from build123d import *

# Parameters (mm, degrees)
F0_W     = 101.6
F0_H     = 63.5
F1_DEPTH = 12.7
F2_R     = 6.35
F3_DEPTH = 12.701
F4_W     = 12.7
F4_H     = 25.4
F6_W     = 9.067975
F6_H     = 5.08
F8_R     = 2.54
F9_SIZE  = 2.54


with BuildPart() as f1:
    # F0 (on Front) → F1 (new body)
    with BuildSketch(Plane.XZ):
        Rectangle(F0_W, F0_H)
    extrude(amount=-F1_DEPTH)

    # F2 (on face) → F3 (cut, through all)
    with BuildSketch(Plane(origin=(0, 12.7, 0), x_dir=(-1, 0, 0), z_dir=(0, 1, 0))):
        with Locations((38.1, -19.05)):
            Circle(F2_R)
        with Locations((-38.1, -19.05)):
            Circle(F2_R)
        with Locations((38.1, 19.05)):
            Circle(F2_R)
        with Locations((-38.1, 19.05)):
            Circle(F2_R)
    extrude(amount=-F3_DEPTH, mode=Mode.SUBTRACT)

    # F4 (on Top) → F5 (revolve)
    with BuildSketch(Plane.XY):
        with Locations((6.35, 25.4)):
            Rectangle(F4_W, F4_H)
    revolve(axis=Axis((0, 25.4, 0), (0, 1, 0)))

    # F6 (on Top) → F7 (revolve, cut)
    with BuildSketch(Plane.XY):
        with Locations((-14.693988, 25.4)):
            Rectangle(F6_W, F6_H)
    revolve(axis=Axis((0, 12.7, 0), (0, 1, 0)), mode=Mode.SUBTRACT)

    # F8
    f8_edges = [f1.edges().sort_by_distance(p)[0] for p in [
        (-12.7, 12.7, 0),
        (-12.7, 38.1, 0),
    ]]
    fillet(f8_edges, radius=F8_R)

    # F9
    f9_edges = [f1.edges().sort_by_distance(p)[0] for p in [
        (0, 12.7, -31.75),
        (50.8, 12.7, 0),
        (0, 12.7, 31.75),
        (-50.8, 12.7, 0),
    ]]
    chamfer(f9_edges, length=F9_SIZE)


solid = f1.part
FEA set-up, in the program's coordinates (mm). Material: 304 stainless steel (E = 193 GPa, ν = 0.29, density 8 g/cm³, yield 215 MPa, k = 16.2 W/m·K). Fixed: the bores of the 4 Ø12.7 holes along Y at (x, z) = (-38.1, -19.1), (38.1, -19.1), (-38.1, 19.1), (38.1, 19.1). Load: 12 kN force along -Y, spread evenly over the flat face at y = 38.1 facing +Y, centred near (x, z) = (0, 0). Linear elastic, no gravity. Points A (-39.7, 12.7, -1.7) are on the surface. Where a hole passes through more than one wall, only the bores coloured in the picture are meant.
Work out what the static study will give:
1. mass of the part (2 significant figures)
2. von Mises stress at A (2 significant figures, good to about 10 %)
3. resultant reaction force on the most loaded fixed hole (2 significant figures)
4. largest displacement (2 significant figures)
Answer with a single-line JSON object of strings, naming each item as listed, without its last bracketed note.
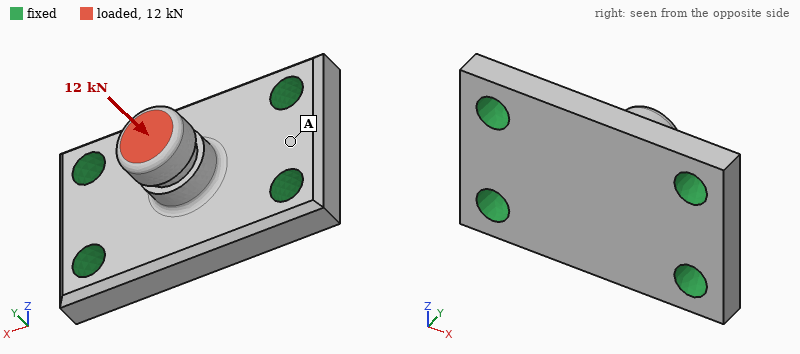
{"mass of the part": "690 g", "von Mises stress at A": "13 MPa", "resultant reaction force on the most loaded fixed hole": "3.1 kN", "largest displacement": "16 µm"}
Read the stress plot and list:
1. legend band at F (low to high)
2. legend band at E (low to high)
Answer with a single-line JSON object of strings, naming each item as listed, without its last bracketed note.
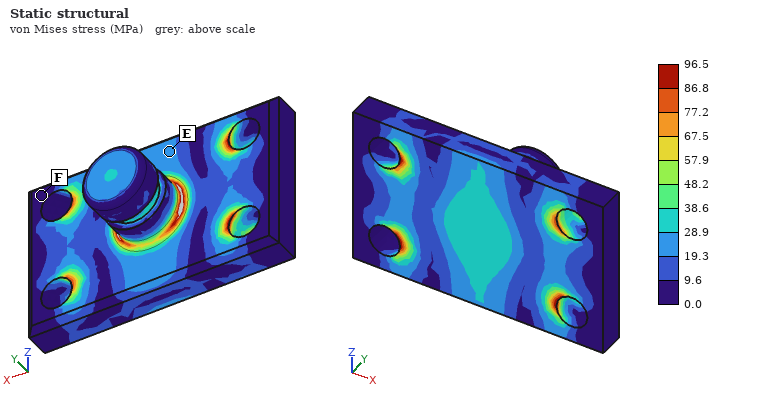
{"legend band at F": "0.0 to 9.6 MPa", "legend band at E": "19.3 to 28.9 MPa"}
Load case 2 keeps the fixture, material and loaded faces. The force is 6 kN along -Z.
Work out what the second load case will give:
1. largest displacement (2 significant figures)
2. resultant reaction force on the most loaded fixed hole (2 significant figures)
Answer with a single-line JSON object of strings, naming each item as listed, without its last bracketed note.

{"largest displacement": "39 µm", "resultant reaction force on the most loaded fixed hole": "3.0 kN"}
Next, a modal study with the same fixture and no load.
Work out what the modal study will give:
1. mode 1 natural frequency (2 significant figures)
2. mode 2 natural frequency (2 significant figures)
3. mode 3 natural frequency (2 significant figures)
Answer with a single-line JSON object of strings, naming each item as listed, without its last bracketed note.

{"mode 1 natural frequency": "9300 Hz", "mode 2 natural frequency": "9600 Hz", "mode 3 natural frequency": "12 kHz"}
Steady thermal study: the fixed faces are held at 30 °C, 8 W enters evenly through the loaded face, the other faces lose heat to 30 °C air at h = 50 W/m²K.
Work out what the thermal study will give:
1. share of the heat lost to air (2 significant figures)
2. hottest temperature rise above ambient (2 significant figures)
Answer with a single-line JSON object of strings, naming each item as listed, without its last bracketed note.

{"share of the heat lost to air": "46 %", "hottest temperature rise above ambient": "35 K"}
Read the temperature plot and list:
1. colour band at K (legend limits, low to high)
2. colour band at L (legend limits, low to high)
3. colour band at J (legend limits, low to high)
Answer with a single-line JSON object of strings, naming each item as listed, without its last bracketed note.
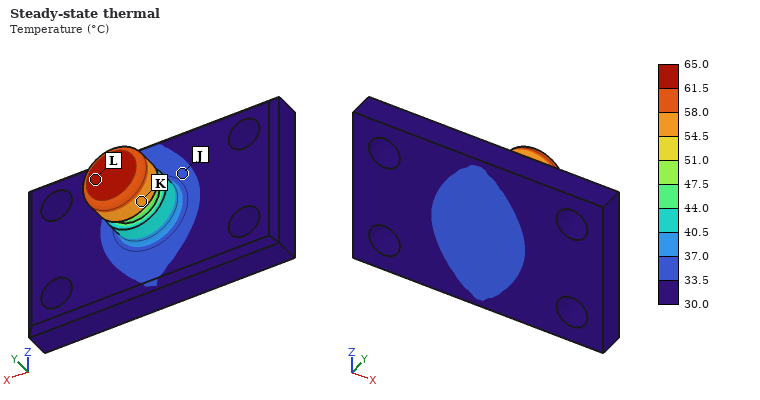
{"colour band at K": "54.5 to 58.0 °C", "colour band at L": "61.5 to 65.0 °C", "colour band at J": "33.5 to 37.0 °C"}
